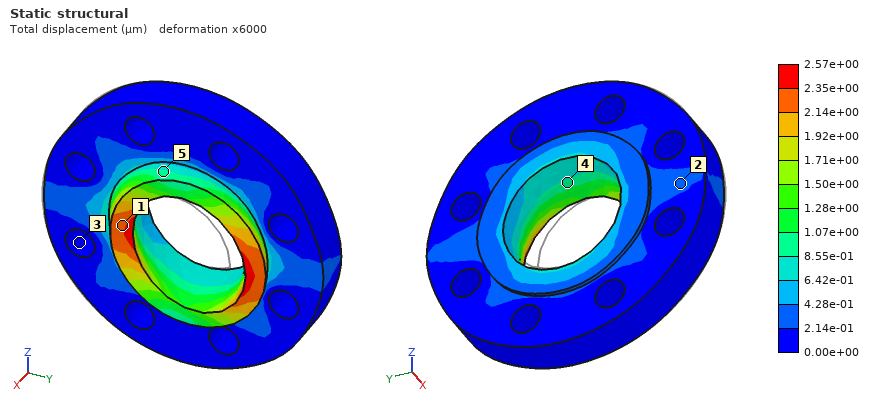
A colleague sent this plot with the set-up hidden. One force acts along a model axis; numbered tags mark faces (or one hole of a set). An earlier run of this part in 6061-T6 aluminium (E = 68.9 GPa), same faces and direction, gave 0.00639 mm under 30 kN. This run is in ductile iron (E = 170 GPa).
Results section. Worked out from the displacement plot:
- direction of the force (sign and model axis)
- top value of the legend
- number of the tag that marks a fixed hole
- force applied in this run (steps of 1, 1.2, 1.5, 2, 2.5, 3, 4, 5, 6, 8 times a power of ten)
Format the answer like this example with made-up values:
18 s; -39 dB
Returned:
+Y; 2.57e+00 µm; 3; 30 kN
